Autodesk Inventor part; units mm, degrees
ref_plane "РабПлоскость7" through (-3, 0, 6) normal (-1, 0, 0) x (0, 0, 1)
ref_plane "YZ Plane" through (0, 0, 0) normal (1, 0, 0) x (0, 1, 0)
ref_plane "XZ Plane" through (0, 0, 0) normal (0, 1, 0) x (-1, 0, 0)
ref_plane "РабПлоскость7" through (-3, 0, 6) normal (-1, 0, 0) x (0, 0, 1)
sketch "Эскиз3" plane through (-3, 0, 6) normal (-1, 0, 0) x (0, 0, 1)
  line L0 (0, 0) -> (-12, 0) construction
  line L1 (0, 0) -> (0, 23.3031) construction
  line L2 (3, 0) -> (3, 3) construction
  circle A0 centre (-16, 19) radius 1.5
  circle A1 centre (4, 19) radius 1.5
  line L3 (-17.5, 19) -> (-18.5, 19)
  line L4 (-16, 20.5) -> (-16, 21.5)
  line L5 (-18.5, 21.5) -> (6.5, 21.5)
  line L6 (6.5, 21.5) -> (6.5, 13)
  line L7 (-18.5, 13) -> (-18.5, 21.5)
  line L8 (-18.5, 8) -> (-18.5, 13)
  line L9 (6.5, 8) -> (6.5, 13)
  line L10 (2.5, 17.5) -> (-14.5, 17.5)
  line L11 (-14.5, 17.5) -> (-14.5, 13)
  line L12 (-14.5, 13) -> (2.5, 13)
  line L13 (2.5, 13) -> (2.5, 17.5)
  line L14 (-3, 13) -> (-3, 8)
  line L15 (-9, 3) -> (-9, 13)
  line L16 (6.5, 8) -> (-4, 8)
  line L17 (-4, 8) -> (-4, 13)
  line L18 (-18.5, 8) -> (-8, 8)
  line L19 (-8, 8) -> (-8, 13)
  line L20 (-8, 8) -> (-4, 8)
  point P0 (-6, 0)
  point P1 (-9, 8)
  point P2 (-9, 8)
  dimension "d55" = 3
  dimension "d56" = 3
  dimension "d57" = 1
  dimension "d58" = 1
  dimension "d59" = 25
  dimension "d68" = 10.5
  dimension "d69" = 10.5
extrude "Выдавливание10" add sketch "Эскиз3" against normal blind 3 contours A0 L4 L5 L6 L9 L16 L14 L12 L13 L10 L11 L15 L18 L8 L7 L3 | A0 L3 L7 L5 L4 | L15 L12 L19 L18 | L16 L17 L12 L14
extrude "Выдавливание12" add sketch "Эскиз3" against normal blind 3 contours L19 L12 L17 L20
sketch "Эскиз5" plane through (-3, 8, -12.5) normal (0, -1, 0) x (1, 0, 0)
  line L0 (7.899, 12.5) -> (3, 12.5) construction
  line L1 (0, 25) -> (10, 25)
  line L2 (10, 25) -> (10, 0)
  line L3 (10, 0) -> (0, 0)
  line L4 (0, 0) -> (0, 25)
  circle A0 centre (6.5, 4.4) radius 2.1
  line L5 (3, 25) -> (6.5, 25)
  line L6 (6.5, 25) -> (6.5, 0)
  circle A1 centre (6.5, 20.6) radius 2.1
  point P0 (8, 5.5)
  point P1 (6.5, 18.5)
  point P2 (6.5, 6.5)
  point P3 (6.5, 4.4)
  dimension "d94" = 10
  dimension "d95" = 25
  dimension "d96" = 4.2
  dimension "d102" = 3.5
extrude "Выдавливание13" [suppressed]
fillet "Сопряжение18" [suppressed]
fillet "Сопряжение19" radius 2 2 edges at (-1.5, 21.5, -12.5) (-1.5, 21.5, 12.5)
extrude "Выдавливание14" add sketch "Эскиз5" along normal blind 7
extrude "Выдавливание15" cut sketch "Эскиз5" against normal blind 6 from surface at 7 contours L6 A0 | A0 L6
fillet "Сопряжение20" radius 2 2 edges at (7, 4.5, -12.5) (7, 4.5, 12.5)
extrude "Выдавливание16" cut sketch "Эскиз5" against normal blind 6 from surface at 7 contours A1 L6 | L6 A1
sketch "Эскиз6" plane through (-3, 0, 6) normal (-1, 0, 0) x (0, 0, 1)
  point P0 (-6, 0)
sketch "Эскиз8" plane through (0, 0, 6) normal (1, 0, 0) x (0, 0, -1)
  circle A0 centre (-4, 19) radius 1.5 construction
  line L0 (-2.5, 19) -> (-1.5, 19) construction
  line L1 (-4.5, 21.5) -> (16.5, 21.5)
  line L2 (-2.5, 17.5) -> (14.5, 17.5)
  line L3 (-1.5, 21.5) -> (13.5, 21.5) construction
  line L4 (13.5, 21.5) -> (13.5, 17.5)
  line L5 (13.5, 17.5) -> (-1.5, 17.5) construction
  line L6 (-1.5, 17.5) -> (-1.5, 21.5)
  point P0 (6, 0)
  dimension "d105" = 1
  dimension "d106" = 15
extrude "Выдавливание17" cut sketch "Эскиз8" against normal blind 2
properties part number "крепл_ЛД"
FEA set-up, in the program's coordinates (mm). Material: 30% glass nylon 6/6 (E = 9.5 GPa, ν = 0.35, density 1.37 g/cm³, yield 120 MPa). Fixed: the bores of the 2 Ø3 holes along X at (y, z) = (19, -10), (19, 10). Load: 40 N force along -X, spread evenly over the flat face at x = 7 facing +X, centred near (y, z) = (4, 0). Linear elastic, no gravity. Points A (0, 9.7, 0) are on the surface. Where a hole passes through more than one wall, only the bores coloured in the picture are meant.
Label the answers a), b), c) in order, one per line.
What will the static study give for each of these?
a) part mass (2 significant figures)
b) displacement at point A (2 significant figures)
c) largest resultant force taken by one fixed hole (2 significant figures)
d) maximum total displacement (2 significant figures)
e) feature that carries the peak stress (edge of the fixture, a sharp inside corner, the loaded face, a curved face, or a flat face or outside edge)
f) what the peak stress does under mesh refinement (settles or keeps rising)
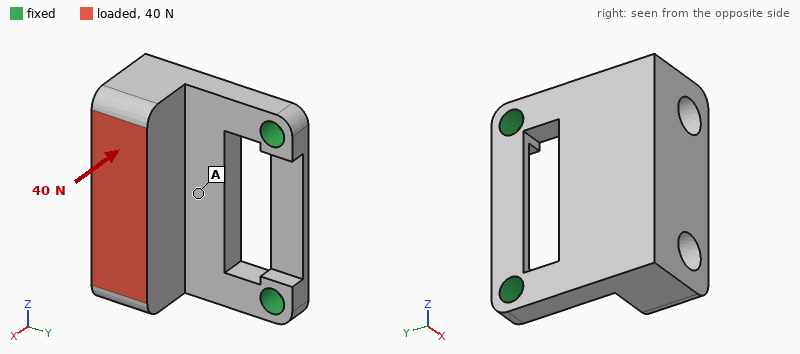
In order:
a) 3.0 g
b) 0.090 mm
c) 20 N
d) 0.28 mm
e) edge of the fixture
f) keeps rising
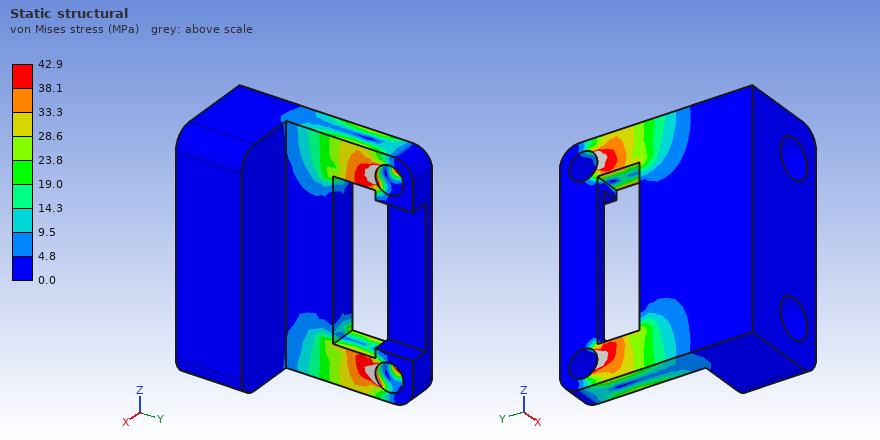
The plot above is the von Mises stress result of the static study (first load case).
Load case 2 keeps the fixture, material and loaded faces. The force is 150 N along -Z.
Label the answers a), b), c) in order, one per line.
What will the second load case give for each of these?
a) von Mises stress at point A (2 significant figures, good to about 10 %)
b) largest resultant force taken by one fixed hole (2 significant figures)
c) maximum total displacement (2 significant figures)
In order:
a) 12 MPa
b) 120 N
c) 0.14 mm
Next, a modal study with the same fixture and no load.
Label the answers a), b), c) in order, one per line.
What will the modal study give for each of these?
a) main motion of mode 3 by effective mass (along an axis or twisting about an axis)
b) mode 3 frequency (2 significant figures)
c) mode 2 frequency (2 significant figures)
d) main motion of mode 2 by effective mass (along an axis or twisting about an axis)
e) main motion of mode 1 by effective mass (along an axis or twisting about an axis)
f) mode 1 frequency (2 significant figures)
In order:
a) along Z
b) 7100 Hz
c) 4700 Hz
d) along Z
e) along X
f) 1400 Hz
